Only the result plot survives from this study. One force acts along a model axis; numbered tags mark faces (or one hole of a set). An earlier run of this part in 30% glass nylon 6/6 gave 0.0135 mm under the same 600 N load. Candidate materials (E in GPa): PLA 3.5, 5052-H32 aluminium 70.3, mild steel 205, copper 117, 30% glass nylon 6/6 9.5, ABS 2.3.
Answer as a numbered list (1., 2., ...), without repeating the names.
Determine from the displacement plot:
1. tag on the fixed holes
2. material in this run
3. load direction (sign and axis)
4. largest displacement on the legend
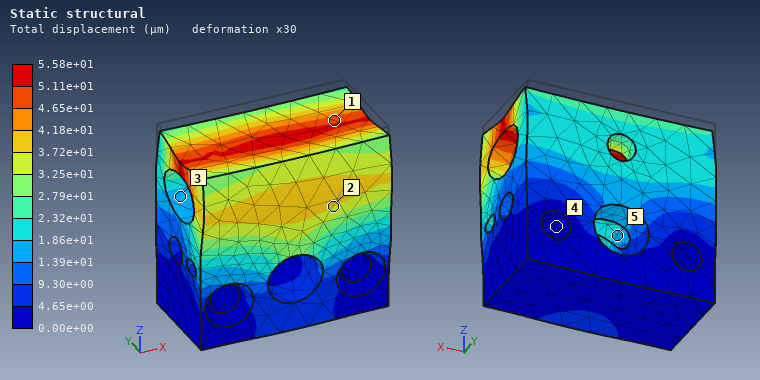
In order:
1. 4
2. ABS
3. -Z
4. 5.58e+01 µm
